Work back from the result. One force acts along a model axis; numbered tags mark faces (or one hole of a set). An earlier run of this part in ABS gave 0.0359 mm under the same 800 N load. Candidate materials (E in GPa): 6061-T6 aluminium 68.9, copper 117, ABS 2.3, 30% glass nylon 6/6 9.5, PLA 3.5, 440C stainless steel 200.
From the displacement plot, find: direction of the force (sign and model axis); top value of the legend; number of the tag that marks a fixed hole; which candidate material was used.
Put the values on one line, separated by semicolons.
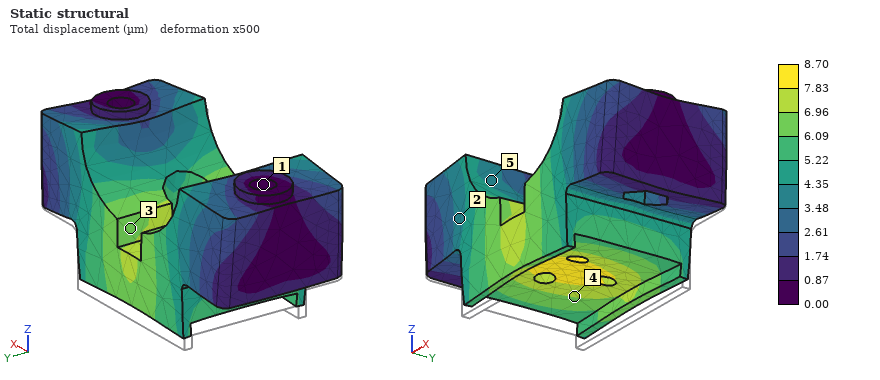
+Z; 8.70 µm; 1; 30% glass nylon 6/6
